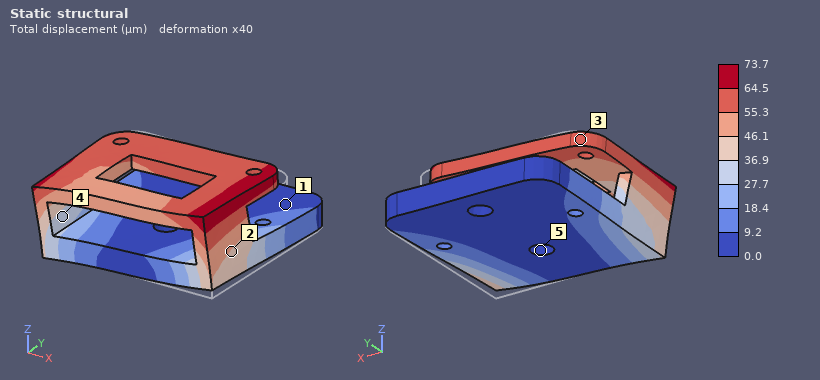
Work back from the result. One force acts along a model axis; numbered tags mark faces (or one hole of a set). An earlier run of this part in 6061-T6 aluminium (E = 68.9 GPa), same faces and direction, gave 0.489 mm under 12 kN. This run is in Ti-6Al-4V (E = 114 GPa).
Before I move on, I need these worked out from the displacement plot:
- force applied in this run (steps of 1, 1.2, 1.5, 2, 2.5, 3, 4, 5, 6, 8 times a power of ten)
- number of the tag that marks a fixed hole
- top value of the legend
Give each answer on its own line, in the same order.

3 kN
5
73.7 µm
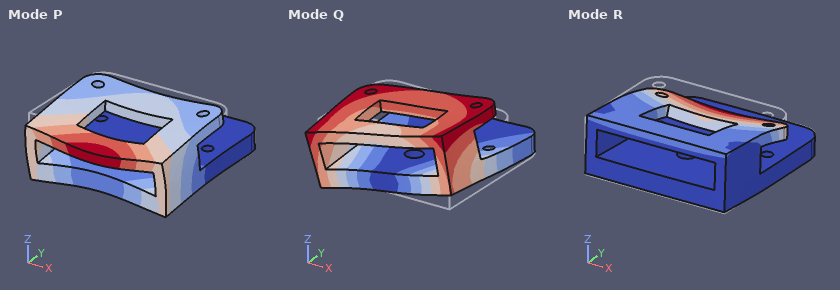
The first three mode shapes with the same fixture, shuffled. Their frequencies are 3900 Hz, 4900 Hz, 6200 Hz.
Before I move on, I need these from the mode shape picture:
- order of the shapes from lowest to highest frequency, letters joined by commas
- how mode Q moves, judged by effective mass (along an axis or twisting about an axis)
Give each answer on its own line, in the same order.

R, Q, P
along X
